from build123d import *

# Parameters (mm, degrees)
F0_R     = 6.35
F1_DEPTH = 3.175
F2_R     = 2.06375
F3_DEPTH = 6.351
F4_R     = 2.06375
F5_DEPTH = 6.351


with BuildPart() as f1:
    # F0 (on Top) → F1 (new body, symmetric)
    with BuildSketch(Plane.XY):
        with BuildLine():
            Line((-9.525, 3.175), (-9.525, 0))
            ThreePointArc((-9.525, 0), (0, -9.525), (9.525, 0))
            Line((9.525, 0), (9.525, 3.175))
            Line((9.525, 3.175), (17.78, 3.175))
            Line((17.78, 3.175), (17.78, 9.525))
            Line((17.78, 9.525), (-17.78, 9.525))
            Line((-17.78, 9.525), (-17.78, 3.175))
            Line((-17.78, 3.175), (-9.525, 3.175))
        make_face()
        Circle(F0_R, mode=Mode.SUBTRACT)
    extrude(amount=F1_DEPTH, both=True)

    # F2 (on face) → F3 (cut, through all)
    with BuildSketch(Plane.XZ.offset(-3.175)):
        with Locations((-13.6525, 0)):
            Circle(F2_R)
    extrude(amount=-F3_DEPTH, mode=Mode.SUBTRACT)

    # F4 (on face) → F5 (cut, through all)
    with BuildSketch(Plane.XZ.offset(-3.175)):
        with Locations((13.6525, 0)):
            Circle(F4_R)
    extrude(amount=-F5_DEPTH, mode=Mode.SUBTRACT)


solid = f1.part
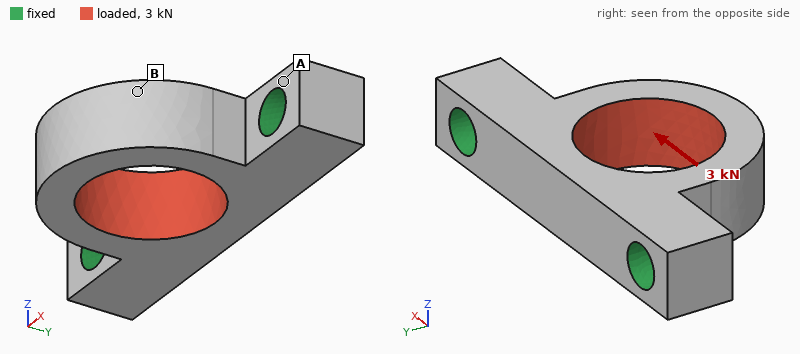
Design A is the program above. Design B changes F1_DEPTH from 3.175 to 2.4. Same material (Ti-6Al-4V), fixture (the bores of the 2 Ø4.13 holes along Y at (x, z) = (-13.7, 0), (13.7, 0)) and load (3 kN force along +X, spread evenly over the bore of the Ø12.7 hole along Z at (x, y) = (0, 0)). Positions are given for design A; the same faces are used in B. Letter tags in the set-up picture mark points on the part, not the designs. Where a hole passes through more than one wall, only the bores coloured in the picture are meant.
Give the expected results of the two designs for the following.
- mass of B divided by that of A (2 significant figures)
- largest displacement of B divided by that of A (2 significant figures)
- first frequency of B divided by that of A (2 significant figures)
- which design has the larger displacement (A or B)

0.73
1.3
0.84
B
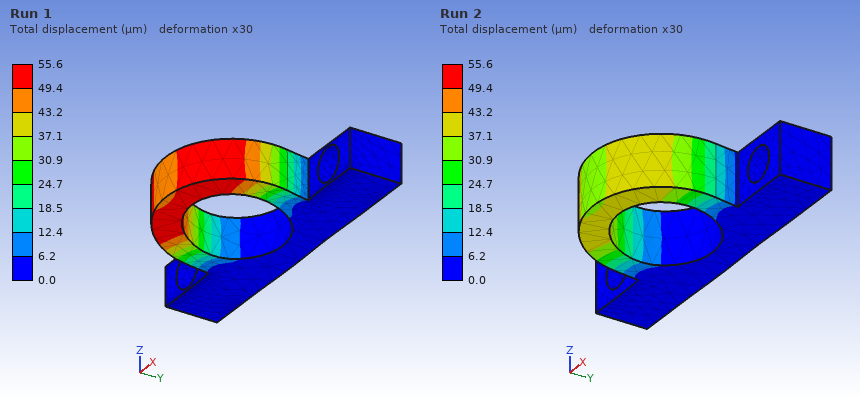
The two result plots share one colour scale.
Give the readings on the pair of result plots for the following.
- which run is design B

Run 1
